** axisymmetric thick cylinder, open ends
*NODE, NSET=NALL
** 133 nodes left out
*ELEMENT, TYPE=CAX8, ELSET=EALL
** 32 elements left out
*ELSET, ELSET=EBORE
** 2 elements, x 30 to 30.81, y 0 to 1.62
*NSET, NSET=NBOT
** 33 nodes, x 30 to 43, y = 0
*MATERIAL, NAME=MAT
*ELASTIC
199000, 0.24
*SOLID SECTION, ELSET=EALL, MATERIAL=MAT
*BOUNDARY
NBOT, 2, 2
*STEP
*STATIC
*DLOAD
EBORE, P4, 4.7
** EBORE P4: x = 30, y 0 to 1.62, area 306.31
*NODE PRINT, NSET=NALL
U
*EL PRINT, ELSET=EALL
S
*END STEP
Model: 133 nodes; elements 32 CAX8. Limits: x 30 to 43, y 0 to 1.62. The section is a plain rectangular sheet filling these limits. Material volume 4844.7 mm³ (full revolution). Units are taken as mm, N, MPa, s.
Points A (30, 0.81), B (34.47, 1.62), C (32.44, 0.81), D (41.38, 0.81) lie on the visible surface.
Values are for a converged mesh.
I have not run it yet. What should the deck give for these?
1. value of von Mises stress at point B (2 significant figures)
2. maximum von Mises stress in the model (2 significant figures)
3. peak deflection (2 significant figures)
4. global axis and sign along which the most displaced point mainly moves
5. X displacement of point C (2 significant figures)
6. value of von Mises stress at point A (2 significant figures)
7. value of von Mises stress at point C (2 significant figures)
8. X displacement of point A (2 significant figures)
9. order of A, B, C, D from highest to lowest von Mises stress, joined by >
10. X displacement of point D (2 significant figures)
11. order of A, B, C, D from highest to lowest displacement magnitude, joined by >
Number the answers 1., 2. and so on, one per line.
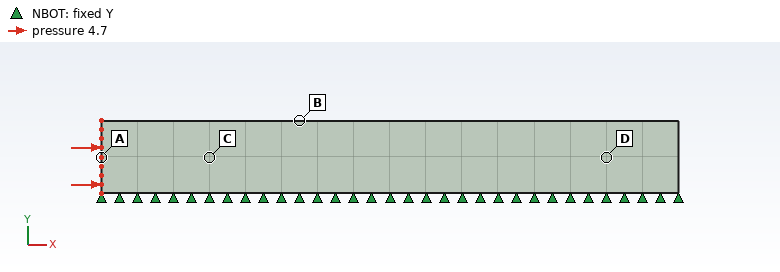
1. 13 MPa
2. 16 MPa
3. 0.0022 mm
4. +X
5. 0.0021 mm
6. 16 MPa
7. 14 MPa
8. 0.0022 mm
9. A > C > B > D
10. 0.0019 mm
11. A > C > B > D
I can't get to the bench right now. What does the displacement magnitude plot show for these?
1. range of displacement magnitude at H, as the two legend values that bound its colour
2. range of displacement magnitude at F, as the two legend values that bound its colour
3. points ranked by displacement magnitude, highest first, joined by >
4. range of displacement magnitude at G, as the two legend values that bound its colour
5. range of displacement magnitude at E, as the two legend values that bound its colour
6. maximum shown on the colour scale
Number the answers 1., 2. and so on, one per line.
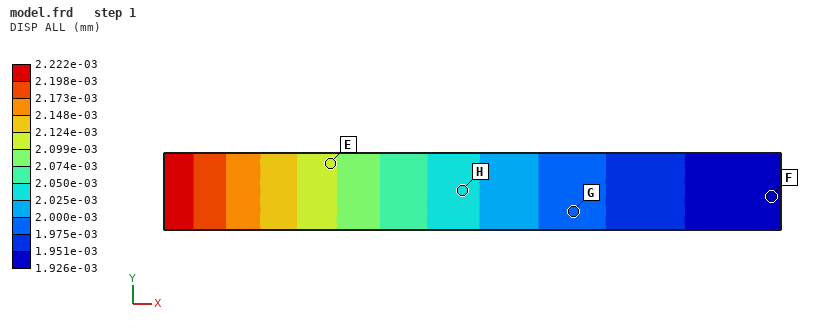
1. 2.025e-03 to 2.050e-03 mm
2. 1.926e-03 to 1.951e-03 mm
3. E > H > G > F
4. 1.975e-03 to 2.000e-03 mm
5. 2.099e-03 to 2.124e-03 mm
6. 2.222e-03 mm
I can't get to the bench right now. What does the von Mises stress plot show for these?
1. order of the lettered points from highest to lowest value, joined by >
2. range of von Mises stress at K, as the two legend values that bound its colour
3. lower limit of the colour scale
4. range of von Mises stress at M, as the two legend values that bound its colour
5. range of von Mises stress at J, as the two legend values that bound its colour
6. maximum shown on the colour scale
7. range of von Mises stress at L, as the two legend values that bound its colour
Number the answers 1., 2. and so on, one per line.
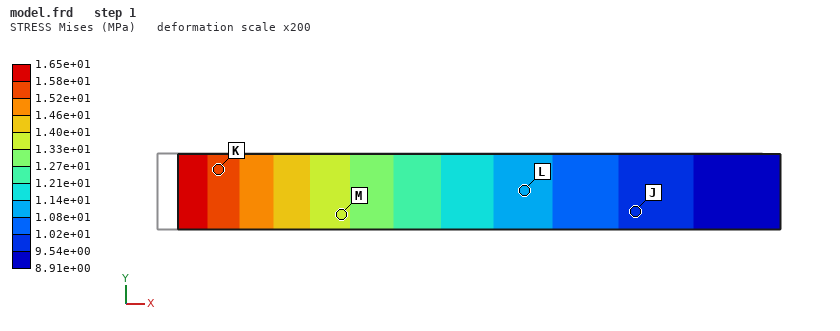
1. K > M > L > J
2. 1.52e+01 to 1.58e+01 MPa
3. 8.91e+00 MPa
4. 1.33e+01 to 1.40e+01 MPa
5. 9.54e+00 to 1.02e+01 MPa
6. 1.65e+01 MPa
7. 1.08e+01 to 1.14e+01 MPa
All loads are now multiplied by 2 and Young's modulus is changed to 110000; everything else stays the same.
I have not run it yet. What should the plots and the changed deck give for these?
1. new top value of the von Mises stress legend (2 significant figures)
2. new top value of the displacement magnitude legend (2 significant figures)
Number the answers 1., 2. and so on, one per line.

1. 33 MPa
2. 0.0080 mm
